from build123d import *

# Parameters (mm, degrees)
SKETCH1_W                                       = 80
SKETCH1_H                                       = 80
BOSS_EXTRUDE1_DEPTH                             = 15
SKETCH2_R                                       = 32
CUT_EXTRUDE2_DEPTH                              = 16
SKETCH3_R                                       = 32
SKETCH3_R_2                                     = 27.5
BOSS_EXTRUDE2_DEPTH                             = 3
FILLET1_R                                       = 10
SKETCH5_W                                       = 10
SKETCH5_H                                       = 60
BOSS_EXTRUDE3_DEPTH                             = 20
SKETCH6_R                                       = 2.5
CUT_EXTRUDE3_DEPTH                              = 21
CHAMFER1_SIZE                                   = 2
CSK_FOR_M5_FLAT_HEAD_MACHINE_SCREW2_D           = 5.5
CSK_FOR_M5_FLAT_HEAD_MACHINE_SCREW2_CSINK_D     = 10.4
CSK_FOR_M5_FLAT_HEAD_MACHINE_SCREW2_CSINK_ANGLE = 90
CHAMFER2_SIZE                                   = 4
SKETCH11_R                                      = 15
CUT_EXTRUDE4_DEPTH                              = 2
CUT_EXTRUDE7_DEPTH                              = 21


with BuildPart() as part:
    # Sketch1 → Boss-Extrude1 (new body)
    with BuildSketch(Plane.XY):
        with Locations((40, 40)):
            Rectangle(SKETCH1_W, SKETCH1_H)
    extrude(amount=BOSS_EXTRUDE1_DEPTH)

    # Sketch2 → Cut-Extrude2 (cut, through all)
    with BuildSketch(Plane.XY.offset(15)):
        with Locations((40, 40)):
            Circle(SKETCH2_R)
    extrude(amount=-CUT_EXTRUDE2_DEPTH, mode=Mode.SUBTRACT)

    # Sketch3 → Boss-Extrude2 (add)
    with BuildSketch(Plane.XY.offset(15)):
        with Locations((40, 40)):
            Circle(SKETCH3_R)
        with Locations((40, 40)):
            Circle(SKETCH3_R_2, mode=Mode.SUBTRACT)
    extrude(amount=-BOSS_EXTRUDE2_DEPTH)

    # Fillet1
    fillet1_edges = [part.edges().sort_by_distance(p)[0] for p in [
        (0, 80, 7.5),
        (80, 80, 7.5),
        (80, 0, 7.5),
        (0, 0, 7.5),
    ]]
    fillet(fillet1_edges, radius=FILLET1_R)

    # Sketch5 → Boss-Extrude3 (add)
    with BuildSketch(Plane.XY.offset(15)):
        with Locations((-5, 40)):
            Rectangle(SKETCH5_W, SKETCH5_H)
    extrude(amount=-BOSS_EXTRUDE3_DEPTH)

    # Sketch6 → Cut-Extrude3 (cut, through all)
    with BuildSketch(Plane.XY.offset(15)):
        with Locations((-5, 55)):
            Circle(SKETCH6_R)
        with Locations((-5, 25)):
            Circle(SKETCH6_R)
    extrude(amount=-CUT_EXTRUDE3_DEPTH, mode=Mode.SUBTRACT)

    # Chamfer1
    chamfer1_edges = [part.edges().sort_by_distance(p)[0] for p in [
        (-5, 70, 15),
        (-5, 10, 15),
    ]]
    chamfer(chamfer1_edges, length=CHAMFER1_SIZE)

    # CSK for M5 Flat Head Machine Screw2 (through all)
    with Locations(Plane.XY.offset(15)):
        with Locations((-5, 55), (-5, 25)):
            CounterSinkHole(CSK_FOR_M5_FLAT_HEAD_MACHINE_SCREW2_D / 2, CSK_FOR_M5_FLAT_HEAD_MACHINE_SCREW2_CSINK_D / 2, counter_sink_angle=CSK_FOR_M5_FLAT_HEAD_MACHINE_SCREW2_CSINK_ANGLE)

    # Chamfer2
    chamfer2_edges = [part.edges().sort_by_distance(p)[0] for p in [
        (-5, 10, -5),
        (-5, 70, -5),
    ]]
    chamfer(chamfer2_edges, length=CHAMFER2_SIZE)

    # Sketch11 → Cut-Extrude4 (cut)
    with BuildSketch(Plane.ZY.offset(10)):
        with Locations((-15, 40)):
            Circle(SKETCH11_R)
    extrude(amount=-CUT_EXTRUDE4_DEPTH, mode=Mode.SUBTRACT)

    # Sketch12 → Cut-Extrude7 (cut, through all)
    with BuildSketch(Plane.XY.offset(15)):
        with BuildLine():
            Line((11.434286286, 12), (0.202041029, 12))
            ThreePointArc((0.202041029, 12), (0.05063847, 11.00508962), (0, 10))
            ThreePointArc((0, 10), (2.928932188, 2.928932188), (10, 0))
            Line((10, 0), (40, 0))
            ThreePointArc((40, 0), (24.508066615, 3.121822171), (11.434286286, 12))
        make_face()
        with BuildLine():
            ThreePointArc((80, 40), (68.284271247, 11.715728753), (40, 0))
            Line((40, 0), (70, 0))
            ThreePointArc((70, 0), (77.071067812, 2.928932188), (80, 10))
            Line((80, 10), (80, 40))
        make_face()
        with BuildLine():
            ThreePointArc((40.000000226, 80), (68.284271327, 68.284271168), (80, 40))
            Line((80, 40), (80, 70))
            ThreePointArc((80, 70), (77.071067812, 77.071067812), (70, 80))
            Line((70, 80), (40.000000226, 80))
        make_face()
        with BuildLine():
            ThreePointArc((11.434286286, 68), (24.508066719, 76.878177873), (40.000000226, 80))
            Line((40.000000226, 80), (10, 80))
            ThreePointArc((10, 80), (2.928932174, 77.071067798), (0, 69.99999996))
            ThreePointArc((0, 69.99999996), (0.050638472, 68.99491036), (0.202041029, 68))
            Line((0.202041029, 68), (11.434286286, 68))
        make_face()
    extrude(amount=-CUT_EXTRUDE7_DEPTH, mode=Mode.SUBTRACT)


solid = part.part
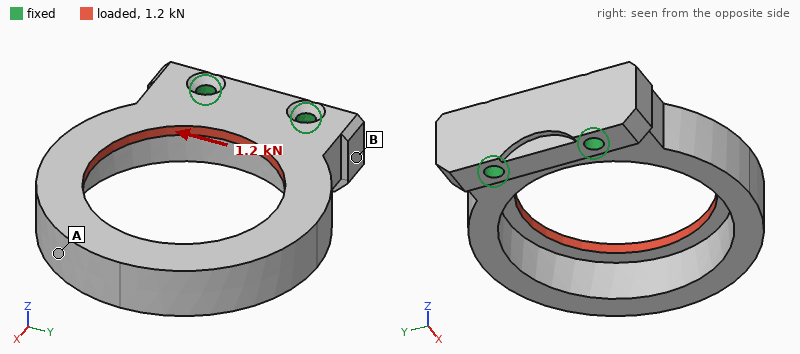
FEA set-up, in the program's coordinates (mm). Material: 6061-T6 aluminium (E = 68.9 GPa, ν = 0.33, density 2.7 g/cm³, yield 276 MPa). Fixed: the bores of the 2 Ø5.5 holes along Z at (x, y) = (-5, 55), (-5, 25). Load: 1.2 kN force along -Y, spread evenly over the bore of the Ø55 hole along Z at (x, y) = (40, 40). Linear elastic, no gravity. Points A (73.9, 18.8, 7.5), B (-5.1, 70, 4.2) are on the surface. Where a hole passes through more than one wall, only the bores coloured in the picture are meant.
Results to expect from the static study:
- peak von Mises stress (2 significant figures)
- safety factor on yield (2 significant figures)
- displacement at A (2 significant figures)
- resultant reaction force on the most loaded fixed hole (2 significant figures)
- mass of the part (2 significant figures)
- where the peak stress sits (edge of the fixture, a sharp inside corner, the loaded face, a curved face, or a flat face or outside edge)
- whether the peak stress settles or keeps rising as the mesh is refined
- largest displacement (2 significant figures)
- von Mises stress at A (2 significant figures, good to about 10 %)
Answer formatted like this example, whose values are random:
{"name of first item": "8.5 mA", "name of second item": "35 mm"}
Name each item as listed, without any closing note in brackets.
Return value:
{"peak von Mises stress": "69 MPa", "safety factor on yield": "4.0", "displacement at A": "0.13 mm", "resultant reaction force on the most loaded fixed hole": "1.5 kN", "mass of the part": "120 g", "where the peak stress sits": "the loaded face", "whether the peak stress settles or keeps rising as the mesh is refined": "settles", "largest displacement": "0.13 mm", "von Mises stress at A": "14 MPa"}
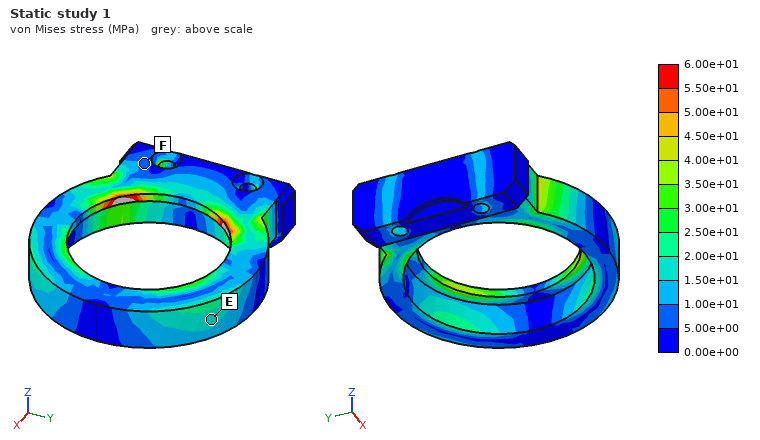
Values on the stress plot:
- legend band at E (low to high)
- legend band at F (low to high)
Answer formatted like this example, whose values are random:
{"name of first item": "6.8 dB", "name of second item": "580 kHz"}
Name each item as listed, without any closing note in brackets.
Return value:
{"legend band at E": "1.50e+01 to 2.00e+01 MPa", "legend band at F": "5.00e+00 to 1.00e+01 MPa"}
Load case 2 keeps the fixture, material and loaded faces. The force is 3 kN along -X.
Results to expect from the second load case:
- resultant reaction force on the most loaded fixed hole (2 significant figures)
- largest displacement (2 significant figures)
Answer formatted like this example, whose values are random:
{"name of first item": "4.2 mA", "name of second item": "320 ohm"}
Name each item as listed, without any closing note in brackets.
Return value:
{"resultant reaction force on the most loaded fixed hole": "1.7 kN", "largest displacement": "0.13 mm"}
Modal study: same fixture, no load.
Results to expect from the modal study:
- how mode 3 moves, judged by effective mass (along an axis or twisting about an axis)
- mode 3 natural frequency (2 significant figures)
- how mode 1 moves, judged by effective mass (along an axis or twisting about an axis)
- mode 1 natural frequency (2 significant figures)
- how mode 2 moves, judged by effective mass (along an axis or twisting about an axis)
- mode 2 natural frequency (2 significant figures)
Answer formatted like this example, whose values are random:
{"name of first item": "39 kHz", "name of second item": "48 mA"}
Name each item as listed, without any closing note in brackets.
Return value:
{"how mode 3 moves, judged by effective mass": "twisting about X", "mode 3 natural frequency": "3300 Hz", "how mode 1 moves, judged by effective mass": "along Z", "mode 1 natural frequency": "1300 Hz", "how mode 2 moves, judged by effective mass": "along Y", "mode 2 natural frequency": "1800 Hz"}
